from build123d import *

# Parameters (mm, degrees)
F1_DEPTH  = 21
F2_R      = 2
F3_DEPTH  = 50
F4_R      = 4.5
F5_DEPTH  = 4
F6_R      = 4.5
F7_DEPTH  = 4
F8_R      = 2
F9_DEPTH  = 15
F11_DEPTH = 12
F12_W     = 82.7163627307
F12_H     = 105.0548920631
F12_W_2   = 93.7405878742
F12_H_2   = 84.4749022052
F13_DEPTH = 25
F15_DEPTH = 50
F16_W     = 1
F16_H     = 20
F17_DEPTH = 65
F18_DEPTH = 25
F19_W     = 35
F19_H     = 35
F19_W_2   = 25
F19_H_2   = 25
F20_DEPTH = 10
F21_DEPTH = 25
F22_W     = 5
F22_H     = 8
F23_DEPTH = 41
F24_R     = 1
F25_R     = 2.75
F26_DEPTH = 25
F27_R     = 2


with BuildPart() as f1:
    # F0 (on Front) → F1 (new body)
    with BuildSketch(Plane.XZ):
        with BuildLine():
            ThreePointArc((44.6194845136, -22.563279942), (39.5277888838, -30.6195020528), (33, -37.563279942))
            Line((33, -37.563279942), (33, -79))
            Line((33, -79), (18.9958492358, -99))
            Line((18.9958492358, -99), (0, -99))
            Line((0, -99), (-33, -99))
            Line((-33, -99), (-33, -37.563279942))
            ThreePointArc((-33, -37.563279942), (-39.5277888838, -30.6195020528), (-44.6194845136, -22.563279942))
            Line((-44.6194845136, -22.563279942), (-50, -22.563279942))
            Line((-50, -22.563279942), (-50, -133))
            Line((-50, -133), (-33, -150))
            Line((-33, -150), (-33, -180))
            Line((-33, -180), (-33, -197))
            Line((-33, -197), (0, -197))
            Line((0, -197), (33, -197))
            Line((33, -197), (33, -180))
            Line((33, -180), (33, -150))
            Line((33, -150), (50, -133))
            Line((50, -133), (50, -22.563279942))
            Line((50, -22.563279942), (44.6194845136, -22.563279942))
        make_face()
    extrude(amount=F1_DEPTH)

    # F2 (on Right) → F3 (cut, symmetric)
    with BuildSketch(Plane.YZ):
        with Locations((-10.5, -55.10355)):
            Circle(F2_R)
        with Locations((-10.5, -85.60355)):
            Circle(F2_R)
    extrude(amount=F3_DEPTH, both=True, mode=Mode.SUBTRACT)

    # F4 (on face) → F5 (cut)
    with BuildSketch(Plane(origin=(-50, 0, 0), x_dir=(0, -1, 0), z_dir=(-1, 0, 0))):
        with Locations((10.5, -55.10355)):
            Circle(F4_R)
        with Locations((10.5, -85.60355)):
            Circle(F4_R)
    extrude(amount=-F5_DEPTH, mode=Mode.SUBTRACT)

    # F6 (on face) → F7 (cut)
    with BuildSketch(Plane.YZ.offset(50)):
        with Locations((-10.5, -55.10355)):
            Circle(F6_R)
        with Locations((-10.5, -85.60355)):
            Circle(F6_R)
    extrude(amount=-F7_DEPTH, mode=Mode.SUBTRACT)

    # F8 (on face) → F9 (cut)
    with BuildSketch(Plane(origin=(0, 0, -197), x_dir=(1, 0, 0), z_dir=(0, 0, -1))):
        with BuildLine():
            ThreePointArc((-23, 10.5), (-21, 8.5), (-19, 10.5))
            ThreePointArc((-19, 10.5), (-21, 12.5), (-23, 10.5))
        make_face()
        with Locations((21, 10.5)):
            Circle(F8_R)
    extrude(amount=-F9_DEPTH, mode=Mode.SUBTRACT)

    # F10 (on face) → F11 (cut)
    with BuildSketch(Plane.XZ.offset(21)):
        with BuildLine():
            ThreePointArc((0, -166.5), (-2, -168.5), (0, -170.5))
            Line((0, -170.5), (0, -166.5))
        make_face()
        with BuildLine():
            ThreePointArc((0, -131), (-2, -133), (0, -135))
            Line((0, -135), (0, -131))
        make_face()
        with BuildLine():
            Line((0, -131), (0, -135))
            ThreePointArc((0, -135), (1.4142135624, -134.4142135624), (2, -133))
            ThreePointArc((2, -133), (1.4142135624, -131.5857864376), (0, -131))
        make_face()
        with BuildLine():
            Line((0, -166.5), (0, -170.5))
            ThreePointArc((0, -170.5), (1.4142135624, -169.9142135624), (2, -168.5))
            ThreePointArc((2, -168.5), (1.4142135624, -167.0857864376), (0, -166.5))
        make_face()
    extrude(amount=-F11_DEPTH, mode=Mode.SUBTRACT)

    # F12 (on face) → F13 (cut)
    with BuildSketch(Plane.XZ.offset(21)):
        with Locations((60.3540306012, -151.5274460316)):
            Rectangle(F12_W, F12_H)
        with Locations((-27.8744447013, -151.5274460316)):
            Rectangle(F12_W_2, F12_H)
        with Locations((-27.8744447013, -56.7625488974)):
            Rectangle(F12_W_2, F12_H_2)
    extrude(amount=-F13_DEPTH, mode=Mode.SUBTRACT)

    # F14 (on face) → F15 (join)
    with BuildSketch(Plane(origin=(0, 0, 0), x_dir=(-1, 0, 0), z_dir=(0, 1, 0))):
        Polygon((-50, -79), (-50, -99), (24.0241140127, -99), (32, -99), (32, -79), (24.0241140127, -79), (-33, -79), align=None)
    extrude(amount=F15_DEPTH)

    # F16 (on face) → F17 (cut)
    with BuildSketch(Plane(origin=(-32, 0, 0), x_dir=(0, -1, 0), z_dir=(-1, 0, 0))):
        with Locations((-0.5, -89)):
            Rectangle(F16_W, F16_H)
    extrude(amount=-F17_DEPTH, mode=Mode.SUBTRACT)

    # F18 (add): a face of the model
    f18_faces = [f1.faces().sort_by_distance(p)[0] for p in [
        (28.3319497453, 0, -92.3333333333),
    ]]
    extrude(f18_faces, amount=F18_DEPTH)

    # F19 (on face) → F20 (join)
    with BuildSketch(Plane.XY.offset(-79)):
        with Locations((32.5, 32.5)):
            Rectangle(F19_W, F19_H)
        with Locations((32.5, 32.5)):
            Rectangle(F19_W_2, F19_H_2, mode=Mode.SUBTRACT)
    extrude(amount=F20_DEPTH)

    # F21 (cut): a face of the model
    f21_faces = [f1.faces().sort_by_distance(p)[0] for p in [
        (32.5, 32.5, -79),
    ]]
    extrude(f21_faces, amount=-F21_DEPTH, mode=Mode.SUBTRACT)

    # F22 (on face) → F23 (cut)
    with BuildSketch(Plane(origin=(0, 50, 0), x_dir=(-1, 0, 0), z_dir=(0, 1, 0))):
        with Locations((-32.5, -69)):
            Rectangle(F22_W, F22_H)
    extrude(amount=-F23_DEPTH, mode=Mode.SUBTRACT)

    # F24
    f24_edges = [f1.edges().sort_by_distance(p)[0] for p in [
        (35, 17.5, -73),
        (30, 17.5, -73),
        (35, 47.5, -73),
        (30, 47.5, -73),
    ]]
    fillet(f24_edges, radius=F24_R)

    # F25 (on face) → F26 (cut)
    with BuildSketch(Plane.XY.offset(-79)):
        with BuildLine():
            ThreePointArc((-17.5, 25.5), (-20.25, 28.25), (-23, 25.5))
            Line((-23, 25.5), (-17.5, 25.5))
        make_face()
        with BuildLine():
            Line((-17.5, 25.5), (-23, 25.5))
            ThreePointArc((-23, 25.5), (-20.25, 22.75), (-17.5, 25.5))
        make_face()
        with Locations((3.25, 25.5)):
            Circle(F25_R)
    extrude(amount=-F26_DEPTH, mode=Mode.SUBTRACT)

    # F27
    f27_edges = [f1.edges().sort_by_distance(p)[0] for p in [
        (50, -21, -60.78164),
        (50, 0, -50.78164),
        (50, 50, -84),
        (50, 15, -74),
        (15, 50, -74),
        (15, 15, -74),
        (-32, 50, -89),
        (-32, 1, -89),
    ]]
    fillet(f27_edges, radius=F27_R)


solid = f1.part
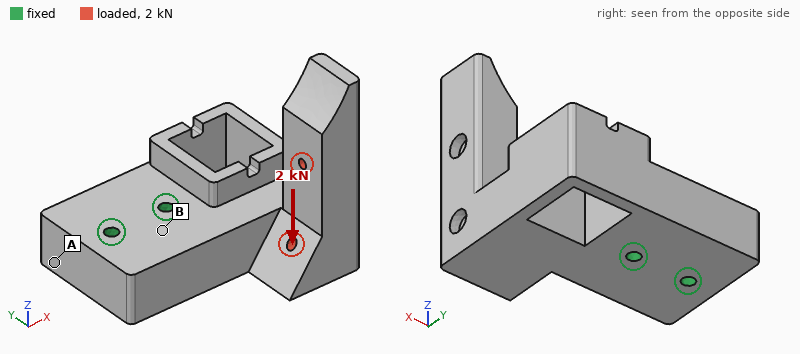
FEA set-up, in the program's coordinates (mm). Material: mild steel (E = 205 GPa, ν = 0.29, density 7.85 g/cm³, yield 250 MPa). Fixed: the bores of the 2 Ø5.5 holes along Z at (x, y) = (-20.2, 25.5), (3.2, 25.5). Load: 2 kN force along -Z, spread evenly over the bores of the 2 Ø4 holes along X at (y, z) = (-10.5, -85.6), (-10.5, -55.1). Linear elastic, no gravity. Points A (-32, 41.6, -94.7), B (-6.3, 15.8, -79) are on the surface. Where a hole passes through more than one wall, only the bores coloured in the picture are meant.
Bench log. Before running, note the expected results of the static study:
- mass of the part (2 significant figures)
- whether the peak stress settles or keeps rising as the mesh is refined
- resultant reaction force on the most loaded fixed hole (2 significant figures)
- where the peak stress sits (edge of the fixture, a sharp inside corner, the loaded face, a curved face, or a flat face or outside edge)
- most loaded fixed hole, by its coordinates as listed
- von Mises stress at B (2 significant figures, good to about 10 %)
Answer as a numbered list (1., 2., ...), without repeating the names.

1. 790 g
2. keeps rising
3. 2.9 kN
4. edge of the fixture
5. (3.2, 25.5)
6. 19 MPa
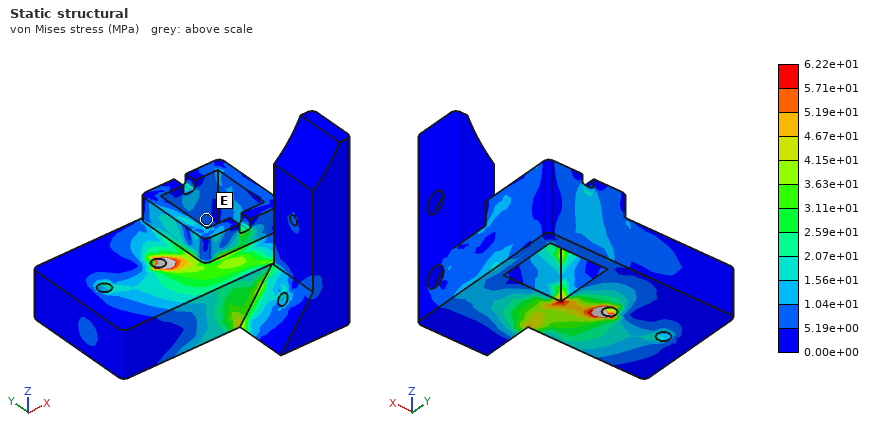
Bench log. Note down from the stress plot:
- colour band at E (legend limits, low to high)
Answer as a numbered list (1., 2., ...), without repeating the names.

1. 5.19e+00 to 1.04e+01 MPa
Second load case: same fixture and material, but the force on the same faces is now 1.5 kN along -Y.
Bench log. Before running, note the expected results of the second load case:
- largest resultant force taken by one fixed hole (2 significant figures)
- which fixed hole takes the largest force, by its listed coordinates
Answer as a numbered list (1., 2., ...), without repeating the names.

1. 3.3 kN
2. (3.2, 25.5)
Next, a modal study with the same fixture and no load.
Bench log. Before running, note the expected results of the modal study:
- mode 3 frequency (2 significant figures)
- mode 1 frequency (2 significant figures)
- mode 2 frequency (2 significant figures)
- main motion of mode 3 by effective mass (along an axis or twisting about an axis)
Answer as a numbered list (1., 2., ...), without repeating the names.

1. 4200 Hz
2. 1800 Hz
3. 2100 Hz
4. along Y
